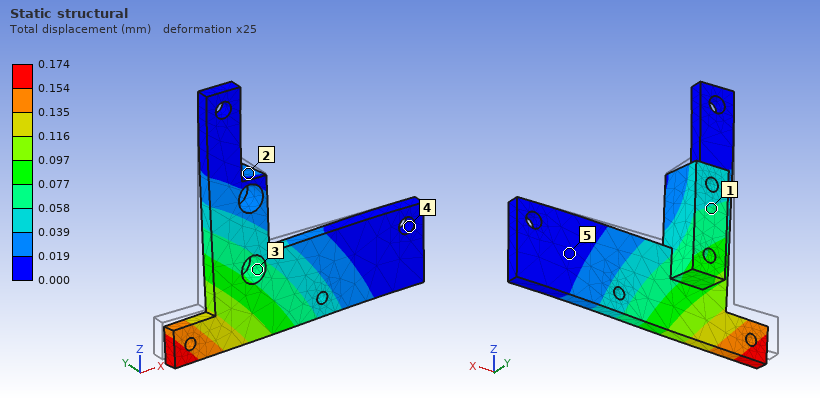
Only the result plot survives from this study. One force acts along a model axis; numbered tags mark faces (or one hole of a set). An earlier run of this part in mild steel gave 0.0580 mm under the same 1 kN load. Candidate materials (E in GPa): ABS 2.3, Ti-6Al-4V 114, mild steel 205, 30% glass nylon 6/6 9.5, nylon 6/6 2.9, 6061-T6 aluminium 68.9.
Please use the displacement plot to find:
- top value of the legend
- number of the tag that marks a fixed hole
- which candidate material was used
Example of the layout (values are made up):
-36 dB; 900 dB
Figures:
0.174 mm; 4; 6061-T6 aluminium
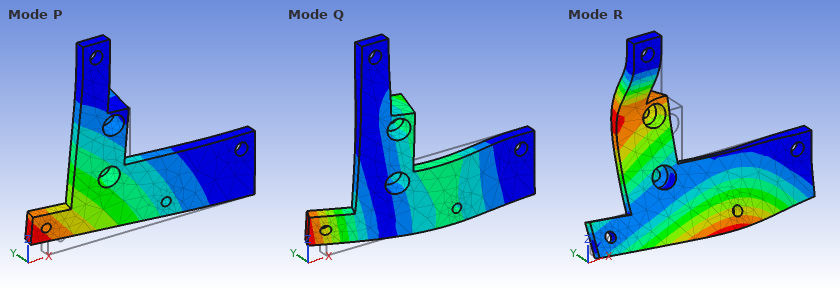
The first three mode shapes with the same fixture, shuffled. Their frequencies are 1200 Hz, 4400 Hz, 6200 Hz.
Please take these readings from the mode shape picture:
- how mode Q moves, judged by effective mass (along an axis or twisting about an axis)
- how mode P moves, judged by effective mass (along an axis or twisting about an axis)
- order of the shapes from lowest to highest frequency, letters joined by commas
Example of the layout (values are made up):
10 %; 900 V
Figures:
along Y; along Y; P, Q, R
